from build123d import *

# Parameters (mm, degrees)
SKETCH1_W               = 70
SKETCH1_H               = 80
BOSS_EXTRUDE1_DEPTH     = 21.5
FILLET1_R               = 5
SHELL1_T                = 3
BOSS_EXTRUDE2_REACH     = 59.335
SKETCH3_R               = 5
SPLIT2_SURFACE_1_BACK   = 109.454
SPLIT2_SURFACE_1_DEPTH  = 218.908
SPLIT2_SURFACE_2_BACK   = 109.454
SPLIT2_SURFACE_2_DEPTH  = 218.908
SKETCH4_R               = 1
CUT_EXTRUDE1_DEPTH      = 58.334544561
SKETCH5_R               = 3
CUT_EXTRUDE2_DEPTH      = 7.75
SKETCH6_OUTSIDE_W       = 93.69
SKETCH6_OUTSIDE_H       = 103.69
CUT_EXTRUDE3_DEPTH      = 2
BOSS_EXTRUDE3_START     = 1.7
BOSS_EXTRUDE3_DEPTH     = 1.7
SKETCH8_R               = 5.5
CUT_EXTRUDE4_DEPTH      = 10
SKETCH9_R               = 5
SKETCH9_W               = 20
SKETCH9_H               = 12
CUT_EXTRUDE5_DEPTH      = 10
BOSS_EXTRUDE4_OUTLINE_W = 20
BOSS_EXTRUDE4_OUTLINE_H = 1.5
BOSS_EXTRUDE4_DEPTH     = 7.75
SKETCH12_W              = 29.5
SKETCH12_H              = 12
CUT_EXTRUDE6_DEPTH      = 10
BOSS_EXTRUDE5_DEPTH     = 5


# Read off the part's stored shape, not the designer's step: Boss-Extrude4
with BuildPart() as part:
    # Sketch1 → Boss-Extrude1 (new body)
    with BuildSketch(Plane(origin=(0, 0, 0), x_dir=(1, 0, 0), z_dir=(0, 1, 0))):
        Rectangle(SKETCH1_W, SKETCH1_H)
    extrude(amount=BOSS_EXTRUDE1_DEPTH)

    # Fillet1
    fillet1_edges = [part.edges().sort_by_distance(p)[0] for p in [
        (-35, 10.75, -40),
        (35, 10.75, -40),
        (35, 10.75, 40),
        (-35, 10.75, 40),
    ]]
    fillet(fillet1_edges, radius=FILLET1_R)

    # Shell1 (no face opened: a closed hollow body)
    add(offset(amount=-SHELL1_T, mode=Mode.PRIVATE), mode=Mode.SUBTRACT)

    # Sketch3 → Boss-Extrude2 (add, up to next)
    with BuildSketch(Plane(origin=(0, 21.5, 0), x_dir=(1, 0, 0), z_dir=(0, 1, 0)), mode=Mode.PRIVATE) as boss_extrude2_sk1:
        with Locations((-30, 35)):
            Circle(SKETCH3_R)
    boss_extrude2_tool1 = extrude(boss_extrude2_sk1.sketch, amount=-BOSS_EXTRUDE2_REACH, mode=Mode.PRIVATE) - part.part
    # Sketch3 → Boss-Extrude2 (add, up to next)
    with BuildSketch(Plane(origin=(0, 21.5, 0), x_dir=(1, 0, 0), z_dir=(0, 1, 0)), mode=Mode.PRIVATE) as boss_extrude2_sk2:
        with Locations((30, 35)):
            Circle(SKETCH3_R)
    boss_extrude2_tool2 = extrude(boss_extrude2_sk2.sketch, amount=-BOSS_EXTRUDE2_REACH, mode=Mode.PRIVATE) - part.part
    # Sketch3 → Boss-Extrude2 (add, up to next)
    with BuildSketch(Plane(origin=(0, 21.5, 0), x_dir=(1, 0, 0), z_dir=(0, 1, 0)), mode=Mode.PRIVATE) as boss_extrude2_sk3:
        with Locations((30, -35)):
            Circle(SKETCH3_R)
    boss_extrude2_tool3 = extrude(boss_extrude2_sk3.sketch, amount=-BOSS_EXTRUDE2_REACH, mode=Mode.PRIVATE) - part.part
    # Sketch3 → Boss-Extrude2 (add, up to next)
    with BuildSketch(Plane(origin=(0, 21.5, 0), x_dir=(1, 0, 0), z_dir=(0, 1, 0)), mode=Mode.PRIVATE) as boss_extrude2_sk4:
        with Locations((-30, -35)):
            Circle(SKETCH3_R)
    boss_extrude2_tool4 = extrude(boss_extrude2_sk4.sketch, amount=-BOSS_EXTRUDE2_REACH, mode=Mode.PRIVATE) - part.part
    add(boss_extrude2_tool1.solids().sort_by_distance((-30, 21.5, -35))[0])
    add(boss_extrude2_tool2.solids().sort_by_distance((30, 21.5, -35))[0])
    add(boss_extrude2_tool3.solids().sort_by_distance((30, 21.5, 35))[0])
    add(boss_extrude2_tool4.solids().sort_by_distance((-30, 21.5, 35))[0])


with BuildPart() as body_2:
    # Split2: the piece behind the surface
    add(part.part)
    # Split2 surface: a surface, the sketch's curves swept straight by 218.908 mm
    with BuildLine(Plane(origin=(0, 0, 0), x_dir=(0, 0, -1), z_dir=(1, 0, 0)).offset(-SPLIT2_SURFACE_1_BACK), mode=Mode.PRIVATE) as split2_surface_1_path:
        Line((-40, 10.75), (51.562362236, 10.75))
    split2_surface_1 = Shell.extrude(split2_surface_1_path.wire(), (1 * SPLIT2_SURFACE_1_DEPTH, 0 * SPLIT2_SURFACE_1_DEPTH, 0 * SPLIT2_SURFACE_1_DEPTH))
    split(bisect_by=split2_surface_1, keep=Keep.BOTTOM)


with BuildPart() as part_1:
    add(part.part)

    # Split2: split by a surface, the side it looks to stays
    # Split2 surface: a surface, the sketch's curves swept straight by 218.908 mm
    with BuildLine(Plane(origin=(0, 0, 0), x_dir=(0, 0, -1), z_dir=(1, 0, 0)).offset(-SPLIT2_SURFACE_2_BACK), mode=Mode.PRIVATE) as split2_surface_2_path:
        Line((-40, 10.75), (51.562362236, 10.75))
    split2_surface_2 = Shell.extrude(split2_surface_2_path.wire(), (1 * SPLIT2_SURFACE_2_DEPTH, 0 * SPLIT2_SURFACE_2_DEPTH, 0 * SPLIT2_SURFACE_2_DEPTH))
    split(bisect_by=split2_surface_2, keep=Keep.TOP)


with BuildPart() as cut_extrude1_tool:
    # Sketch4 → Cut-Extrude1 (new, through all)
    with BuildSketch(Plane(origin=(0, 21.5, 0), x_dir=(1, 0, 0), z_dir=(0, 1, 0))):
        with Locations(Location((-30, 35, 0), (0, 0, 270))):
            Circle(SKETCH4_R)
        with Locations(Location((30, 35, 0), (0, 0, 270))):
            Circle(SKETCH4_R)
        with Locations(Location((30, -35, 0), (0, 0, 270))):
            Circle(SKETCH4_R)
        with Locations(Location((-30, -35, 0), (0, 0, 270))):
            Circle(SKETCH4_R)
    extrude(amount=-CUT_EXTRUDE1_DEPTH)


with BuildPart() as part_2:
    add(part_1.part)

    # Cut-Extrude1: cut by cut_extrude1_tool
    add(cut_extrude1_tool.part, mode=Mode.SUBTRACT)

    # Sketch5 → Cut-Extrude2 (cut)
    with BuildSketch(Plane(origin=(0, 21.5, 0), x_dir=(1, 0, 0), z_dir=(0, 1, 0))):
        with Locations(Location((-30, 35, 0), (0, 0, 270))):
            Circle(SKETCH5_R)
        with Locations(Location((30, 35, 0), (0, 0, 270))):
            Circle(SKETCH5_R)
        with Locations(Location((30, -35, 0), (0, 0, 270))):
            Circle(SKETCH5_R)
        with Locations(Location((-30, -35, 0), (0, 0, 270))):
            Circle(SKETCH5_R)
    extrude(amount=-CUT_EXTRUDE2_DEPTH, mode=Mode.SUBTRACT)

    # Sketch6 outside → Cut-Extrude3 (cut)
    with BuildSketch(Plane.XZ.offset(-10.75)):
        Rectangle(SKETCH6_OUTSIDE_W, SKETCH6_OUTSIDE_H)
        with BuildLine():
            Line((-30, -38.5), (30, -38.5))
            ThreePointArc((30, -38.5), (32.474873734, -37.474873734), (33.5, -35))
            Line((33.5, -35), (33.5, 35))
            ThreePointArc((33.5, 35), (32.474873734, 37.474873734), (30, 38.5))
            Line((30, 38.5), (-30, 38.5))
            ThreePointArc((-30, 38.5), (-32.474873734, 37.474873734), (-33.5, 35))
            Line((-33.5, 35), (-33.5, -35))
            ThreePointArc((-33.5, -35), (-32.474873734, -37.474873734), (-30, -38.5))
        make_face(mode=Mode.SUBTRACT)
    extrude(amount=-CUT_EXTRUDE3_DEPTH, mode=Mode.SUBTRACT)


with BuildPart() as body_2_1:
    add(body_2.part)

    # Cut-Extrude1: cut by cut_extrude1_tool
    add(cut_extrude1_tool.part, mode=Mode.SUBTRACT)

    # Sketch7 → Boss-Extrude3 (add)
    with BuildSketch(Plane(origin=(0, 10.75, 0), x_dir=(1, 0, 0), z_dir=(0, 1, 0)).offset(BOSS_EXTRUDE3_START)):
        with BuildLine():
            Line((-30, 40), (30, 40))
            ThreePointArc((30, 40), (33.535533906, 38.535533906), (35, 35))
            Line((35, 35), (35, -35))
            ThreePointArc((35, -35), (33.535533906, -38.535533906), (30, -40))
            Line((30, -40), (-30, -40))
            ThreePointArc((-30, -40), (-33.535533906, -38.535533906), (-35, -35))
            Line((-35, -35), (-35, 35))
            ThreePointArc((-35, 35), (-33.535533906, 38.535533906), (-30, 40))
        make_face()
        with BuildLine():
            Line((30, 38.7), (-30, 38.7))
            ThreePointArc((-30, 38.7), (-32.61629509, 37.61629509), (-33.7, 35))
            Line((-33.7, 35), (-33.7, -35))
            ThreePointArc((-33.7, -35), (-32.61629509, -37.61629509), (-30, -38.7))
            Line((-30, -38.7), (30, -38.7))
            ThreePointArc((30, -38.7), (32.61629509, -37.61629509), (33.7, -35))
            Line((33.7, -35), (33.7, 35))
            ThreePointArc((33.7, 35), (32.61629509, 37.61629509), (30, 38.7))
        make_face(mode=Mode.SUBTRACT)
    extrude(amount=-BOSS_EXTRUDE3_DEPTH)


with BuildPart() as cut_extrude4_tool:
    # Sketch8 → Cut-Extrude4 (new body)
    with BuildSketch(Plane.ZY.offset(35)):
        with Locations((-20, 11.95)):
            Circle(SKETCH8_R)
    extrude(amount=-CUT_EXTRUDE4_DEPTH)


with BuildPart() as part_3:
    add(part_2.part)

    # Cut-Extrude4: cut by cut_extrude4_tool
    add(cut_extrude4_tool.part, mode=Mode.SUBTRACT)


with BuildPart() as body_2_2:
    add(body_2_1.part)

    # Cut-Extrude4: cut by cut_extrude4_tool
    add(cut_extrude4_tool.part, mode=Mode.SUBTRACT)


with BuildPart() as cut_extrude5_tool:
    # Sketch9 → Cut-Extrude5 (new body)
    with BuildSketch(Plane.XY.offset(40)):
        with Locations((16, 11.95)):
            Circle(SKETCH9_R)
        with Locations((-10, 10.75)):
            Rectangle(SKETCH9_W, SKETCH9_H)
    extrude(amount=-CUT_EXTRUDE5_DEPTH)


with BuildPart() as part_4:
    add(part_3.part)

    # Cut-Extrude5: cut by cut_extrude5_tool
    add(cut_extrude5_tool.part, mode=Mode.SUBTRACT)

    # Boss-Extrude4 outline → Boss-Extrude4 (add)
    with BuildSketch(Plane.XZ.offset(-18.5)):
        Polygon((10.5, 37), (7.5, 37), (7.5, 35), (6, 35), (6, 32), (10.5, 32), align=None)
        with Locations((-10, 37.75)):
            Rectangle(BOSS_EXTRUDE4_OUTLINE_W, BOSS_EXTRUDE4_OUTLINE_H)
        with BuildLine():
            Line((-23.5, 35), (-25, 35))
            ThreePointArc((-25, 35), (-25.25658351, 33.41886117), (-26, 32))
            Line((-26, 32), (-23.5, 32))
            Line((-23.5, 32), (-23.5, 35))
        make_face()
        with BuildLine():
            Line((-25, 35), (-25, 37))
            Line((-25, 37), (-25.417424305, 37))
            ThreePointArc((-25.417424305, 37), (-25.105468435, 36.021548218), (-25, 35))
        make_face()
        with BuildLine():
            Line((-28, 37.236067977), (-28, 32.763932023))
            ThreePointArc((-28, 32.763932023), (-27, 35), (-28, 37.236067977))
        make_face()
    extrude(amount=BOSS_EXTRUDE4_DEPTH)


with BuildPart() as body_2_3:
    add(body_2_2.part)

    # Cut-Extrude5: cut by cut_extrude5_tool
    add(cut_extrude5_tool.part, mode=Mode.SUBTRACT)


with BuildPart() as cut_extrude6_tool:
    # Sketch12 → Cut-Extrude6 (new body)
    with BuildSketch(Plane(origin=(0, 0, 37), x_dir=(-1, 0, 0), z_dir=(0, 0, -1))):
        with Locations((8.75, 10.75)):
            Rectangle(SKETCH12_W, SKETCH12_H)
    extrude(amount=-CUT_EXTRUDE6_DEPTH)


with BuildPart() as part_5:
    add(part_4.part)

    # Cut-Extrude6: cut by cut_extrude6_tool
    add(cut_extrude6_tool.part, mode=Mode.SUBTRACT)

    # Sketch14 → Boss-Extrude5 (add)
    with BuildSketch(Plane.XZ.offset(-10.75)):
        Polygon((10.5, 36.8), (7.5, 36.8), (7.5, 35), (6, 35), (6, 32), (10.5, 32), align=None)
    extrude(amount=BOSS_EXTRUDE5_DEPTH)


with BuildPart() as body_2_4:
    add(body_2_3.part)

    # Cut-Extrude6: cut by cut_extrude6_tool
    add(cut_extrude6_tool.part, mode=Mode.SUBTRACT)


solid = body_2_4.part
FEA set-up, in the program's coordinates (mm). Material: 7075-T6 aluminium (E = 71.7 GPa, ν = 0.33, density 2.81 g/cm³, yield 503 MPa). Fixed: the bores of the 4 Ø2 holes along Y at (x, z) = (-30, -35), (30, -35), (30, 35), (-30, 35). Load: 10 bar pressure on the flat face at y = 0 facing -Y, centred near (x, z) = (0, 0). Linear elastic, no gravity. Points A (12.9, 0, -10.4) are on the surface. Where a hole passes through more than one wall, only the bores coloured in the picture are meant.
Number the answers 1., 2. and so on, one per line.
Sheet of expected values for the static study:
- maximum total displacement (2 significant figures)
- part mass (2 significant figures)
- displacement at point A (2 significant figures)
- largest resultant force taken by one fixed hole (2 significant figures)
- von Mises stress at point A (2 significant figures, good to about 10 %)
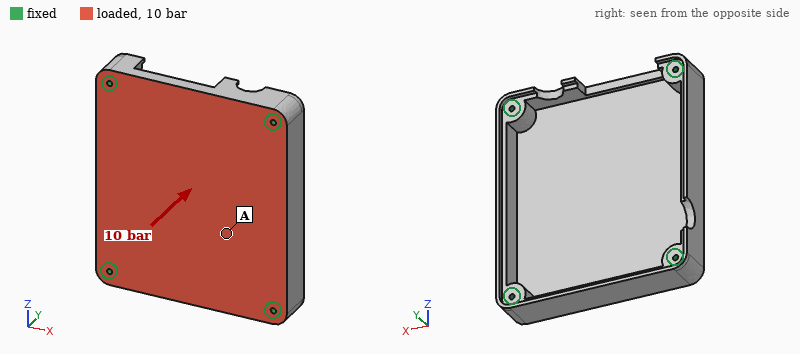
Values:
1. 0.39 mm
2. 68 g
3. 0.29 mm
4. 1.8 kN
5. 92 MPa
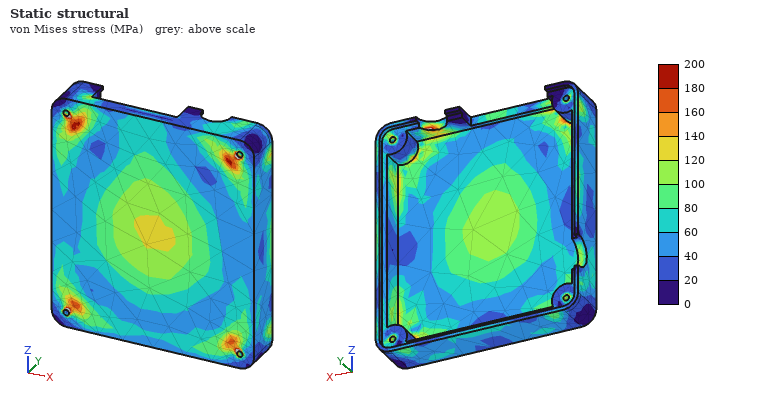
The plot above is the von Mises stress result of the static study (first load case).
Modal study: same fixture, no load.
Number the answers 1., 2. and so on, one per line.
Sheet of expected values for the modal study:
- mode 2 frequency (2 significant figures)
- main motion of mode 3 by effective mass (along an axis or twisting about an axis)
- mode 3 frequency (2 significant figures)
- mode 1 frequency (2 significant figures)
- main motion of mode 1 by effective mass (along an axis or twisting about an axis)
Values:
1. 6800 Hz
2. twisting about Z
3. 7200 Hz
4. 3400 Hz
5. along Y
